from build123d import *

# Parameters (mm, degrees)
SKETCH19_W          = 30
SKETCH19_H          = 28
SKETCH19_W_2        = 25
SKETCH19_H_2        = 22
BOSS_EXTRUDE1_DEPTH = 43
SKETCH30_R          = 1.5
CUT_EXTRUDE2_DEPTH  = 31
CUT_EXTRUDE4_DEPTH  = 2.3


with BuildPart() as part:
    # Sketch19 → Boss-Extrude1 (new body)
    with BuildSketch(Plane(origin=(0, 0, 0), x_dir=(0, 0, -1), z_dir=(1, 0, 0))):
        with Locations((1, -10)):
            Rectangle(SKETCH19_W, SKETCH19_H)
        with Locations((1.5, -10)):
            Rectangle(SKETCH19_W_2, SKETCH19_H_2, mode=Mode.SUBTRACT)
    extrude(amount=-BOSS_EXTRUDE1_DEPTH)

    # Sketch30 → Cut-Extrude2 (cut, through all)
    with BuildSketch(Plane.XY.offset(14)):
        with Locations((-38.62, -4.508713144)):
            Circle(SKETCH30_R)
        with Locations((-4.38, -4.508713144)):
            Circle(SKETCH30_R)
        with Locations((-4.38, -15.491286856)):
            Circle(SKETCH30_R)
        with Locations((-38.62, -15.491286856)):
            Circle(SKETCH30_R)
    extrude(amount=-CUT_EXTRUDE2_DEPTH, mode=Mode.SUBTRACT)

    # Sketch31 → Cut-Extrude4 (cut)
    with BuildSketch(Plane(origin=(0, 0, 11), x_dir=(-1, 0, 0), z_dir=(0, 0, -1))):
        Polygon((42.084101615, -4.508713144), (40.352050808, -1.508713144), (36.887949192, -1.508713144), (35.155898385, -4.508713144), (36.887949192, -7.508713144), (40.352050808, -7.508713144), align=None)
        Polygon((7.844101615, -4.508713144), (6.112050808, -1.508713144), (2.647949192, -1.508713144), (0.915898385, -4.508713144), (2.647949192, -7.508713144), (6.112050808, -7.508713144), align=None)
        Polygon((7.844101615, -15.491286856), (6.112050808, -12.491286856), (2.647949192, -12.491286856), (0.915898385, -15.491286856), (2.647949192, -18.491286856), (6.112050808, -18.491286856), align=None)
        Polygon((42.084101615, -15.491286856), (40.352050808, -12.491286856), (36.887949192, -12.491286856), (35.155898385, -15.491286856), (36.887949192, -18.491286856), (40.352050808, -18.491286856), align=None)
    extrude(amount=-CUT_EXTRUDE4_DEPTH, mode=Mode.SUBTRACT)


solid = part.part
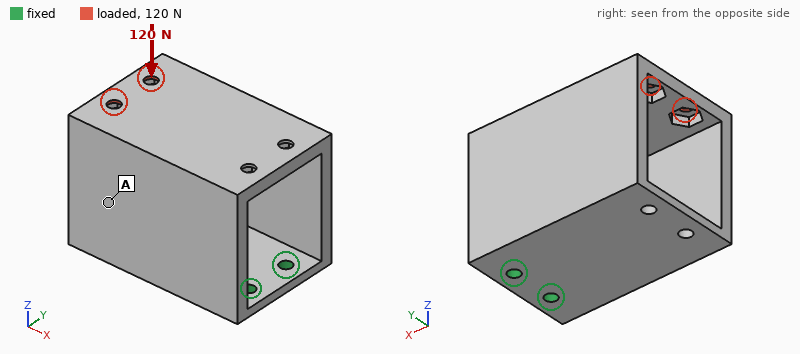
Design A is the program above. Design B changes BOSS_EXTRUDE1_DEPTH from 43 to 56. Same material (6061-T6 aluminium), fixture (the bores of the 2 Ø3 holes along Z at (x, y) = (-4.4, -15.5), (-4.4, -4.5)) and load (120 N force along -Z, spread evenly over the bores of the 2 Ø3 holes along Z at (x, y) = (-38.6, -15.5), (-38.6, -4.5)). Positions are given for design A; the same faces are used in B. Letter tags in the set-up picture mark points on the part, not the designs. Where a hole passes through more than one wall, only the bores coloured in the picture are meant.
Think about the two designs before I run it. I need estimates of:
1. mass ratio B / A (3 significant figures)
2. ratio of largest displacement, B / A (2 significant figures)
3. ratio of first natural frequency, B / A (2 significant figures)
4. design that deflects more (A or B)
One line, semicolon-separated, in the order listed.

1.31; 1.2; 0.72; B
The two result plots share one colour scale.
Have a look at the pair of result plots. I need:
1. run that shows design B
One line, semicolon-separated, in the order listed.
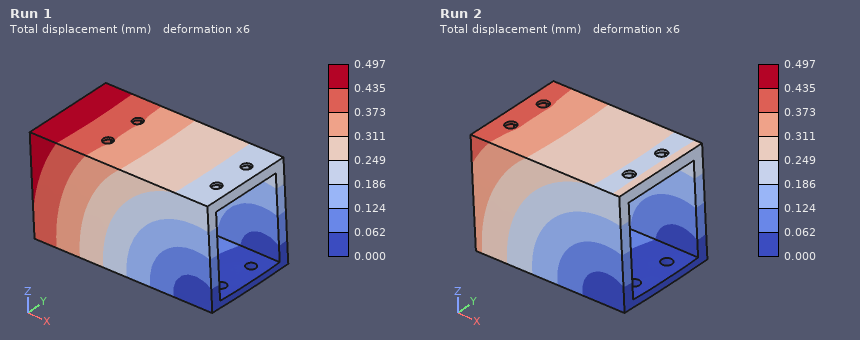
Run 1
